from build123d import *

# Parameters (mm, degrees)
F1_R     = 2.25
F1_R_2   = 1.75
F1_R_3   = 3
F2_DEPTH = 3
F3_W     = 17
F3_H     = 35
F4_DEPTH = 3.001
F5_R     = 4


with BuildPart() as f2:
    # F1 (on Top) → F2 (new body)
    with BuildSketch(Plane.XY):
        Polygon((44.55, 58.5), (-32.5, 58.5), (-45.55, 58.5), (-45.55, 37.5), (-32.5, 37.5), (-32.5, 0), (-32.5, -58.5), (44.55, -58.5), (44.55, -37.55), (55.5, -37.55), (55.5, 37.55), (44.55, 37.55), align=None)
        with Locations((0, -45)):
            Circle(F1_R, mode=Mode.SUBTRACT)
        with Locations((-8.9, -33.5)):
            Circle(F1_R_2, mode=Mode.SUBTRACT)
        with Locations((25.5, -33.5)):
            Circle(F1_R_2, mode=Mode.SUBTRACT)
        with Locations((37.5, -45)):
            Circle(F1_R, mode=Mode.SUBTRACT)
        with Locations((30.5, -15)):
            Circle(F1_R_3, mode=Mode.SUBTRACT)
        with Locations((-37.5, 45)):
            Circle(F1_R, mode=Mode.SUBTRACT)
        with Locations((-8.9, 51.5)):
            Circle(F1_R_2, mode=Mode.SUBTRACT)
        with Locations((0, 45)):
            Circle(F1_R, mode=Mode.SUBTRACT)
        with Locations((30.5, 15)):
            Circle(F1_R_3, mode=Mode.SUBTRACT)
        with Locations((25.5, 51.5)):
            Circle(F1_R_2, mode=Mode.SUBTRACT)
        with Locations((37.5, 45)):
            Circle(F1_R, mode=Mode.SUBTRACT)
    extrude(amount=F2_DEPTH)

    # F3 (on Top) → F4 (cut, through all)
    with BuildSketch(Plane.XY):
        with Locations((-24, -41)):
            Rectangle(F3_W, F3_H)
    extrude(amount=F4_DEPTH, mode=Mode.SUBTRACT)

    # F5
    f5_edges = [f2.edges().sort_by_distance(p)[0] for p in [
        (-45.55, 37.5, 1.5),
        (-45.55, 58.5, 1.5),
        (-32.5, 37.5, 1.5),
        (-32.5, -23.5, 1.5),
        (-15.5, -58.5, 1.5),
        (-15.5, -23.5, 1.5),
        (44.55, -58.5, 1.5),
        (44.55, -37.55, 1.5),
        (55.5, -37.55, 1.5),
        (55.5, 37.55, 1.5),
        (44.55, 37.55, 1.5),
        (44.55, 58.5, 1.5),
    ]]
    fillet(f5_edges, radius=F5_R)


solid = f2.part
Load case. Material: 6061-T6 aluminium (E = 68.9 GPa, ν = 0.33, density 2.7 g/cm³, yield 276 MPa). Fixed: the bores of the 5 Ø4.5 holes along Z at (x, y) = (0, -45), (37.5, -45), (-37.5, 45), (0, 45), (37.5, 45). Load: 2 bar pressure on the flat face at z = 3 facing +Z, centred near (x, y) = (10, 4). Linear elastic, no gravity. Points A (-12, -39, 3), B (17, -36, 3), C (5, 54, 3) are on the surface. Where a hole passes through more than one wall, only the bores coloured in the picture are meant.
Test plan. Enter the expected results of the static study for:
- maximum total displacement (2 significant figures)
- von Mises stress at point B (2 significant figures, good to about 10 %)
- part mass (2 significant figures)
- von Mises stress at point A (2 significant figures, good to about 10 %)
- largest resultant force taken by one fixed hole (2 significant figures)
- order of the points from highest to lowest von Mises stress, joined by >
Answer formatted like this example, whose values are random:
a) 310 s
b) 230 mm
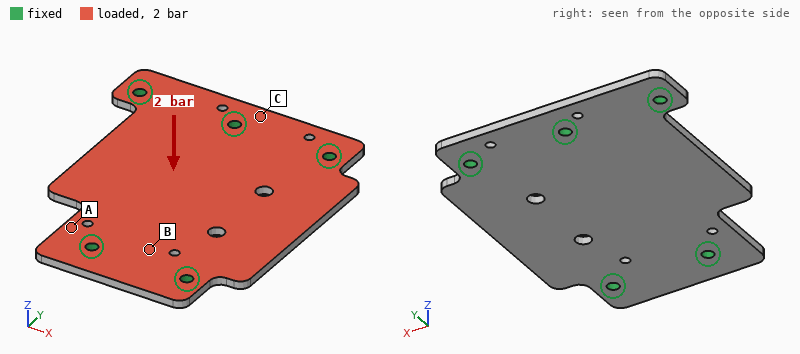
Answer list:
a) 0.36 mm
b) 34 MPa
c) 76 g
d) 56 MPa
e) 470 N
f) A > B > C
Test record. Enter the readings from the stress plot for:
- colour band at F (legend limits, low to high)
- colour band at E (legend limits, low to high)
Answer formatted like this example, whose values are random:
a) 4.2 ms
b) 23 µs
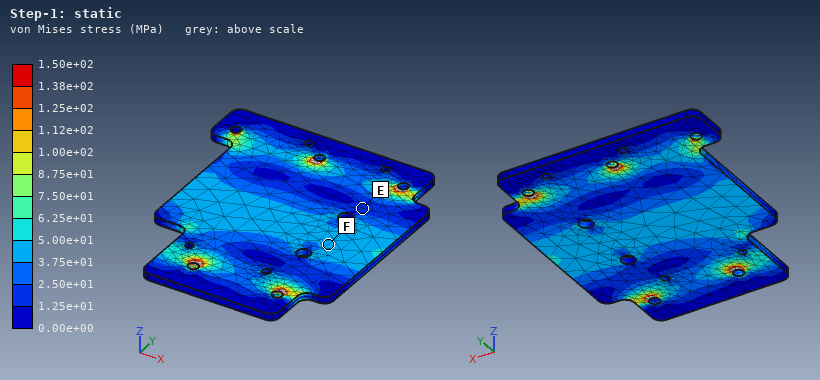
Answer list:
a) 3.75e+01 to 5.00e+01 MPa
b) 1.25e+01 to 2.50e+01 MPa
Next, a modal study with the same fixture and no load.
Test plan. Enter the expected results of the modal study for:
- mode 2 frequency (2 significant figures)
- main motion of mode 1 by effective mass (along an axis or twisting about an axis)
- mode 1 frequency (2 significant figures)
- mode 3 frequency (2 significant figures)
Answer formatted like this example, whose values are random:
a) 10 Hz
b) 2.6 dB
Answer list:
a) 1900 Hz
b) along Z
c) 1700 Hz
d) 3300 Hz
